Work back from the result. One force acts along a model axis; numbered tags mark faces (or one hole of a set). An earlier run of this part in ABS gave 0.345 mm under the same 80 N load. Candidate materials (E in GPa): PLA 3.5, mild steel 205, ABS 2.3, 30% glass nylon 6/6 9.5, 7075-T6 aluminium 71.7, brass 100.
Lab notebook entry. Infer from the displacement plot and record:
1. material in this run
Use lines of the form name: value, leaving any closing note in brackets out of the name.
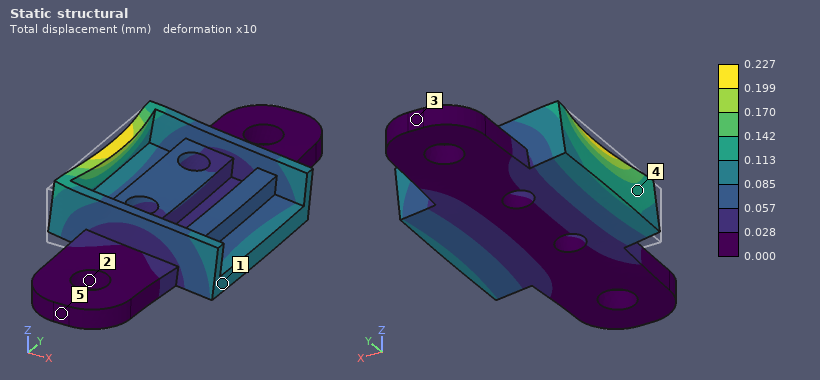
material in this run: PLA
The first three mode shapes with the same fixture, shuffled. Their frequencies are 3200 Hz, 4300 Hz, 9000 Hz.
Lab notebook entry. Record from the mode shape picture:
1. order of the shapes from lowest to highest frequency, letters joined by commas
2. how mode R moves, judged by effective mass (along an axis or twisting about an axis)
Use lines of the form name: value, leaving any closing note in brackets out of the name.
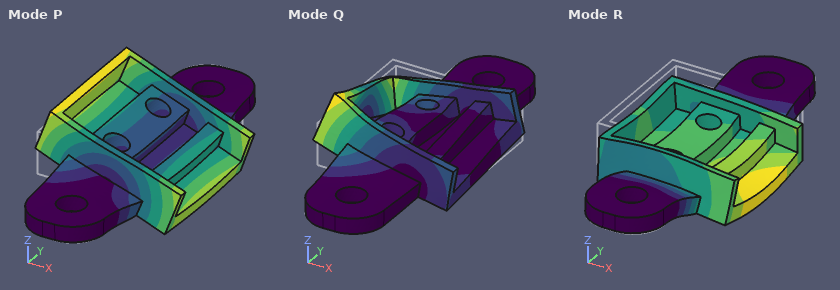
order of the shapes from lowest to highest frequency, letters joined by commas: P, R, Q
how mode R moves, judged by effective mass: along Z
